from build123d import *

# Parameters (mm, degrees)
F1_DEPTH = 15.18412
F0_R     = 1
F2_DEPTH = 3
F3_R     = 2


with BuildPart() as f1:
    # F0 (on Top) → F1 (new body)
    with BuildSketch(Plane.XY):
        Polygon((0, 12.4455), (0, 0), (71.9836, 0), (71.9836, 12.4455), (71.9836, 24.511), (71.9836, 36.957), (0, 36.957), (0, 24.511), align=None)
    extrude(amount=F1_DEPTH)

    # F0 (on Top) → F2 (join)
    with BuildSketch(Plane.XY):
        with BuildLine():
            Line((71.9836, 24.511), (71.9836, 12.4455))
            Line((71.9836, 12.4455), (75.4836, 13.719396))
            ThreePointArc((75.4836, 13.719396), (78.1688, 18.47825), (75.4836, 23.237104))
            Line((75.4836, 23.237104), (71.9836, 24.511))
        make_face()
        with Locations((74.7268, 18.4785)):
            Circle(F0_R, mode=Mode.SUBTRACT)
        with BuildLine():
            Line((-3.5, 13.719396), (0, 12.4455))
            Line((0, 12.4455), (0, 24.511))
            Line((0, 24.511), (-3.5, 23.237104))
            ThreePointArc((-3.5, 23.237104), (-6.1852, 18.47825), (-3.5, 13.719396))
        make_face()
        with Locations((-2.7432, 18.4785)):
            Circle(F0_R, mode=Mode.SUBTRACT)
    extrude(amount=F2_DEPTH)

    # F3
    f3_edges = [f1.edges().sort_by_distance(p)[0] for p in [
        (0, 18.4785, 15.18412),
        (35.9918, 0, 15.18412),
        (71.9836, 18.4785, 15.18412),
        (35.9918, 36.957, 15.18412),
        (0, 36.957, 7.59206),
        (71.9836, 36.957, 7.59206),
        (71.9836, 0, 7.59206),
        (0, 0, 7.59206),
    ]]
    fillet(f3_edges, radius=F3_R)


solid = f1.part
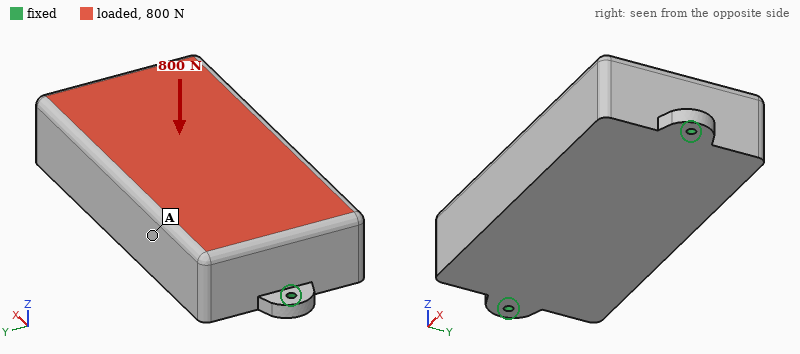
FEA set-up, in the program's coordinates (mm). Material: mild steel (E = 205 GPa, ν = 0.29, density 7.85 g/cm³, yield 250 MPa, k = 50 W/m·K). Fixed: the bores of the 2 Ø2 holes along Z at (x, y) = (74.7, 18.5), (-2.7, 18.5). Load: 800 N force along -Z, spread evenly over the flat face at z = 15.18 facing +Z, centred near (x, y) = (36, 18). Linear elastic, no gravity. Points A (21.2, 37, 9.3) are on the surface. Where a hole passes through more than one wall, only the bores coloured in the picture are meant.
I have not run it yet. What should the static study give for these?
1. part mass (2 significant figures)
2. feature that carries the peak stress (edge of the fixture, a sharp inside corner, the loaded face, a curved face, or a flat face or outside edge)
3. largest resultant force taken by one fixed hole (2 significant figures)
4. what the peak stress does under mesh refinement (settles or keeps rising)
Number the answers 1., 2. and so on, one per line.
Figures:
1. 320 g
2. edge of the fixture
3. 510 N
4. keeps rising
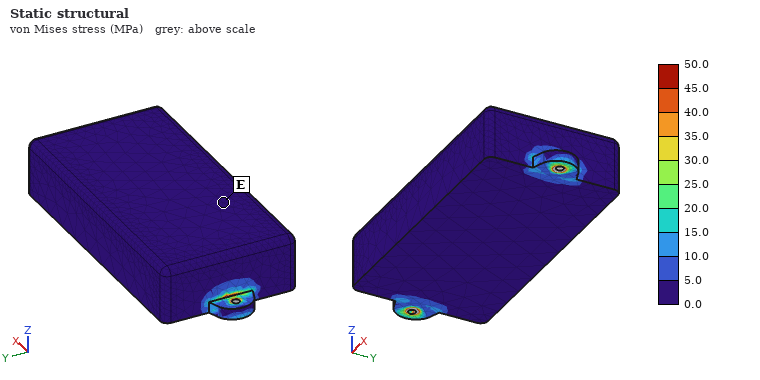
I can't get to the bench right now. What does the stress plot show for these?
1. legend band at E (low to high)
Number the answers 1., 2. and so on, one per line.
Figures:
1. 0.0 to 5.0 MPa
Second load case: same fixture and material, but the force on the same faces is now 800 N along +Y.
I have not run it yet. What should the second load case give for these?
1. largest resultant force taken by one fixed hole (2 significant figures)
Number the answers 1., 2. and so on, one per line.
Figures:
1. 400 N
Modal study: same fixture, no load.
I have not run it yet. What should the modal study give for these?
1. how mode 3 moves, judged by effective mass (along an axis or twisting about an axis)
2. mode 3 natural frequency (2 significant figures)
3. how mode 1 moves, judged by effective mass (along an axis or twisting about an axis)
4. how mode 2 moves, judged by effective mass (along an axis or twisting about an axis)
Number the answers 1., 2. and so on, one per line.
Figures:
1. along Y
2. 8000 Hz
3. along Y
4. along Z
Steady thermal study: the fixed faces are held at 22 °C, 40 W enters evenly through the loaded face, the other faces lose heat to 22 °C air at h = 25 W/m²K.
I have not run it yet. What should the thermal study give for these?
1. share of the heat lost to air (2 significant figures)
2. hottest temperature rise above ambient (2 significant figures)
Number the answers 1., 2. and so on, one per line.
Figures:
1. 24 %
2. 70 K
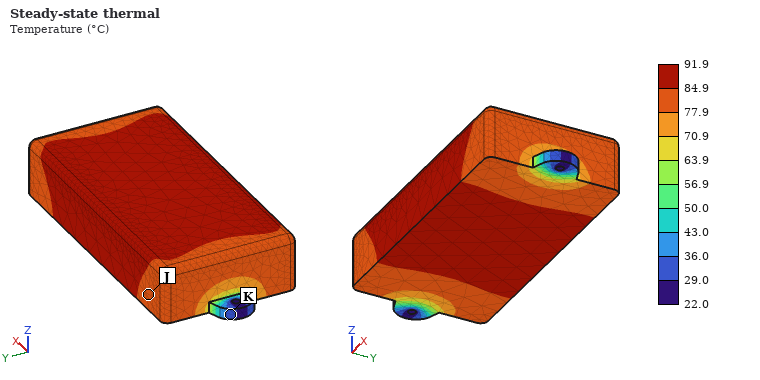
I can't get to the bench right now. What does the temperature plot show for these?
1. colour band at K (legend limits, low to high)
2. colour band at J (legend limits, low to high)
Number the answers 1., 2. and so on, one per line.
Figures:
1. 29.0 to 36.0 °C
2. 77.9 to 84.9 °C
